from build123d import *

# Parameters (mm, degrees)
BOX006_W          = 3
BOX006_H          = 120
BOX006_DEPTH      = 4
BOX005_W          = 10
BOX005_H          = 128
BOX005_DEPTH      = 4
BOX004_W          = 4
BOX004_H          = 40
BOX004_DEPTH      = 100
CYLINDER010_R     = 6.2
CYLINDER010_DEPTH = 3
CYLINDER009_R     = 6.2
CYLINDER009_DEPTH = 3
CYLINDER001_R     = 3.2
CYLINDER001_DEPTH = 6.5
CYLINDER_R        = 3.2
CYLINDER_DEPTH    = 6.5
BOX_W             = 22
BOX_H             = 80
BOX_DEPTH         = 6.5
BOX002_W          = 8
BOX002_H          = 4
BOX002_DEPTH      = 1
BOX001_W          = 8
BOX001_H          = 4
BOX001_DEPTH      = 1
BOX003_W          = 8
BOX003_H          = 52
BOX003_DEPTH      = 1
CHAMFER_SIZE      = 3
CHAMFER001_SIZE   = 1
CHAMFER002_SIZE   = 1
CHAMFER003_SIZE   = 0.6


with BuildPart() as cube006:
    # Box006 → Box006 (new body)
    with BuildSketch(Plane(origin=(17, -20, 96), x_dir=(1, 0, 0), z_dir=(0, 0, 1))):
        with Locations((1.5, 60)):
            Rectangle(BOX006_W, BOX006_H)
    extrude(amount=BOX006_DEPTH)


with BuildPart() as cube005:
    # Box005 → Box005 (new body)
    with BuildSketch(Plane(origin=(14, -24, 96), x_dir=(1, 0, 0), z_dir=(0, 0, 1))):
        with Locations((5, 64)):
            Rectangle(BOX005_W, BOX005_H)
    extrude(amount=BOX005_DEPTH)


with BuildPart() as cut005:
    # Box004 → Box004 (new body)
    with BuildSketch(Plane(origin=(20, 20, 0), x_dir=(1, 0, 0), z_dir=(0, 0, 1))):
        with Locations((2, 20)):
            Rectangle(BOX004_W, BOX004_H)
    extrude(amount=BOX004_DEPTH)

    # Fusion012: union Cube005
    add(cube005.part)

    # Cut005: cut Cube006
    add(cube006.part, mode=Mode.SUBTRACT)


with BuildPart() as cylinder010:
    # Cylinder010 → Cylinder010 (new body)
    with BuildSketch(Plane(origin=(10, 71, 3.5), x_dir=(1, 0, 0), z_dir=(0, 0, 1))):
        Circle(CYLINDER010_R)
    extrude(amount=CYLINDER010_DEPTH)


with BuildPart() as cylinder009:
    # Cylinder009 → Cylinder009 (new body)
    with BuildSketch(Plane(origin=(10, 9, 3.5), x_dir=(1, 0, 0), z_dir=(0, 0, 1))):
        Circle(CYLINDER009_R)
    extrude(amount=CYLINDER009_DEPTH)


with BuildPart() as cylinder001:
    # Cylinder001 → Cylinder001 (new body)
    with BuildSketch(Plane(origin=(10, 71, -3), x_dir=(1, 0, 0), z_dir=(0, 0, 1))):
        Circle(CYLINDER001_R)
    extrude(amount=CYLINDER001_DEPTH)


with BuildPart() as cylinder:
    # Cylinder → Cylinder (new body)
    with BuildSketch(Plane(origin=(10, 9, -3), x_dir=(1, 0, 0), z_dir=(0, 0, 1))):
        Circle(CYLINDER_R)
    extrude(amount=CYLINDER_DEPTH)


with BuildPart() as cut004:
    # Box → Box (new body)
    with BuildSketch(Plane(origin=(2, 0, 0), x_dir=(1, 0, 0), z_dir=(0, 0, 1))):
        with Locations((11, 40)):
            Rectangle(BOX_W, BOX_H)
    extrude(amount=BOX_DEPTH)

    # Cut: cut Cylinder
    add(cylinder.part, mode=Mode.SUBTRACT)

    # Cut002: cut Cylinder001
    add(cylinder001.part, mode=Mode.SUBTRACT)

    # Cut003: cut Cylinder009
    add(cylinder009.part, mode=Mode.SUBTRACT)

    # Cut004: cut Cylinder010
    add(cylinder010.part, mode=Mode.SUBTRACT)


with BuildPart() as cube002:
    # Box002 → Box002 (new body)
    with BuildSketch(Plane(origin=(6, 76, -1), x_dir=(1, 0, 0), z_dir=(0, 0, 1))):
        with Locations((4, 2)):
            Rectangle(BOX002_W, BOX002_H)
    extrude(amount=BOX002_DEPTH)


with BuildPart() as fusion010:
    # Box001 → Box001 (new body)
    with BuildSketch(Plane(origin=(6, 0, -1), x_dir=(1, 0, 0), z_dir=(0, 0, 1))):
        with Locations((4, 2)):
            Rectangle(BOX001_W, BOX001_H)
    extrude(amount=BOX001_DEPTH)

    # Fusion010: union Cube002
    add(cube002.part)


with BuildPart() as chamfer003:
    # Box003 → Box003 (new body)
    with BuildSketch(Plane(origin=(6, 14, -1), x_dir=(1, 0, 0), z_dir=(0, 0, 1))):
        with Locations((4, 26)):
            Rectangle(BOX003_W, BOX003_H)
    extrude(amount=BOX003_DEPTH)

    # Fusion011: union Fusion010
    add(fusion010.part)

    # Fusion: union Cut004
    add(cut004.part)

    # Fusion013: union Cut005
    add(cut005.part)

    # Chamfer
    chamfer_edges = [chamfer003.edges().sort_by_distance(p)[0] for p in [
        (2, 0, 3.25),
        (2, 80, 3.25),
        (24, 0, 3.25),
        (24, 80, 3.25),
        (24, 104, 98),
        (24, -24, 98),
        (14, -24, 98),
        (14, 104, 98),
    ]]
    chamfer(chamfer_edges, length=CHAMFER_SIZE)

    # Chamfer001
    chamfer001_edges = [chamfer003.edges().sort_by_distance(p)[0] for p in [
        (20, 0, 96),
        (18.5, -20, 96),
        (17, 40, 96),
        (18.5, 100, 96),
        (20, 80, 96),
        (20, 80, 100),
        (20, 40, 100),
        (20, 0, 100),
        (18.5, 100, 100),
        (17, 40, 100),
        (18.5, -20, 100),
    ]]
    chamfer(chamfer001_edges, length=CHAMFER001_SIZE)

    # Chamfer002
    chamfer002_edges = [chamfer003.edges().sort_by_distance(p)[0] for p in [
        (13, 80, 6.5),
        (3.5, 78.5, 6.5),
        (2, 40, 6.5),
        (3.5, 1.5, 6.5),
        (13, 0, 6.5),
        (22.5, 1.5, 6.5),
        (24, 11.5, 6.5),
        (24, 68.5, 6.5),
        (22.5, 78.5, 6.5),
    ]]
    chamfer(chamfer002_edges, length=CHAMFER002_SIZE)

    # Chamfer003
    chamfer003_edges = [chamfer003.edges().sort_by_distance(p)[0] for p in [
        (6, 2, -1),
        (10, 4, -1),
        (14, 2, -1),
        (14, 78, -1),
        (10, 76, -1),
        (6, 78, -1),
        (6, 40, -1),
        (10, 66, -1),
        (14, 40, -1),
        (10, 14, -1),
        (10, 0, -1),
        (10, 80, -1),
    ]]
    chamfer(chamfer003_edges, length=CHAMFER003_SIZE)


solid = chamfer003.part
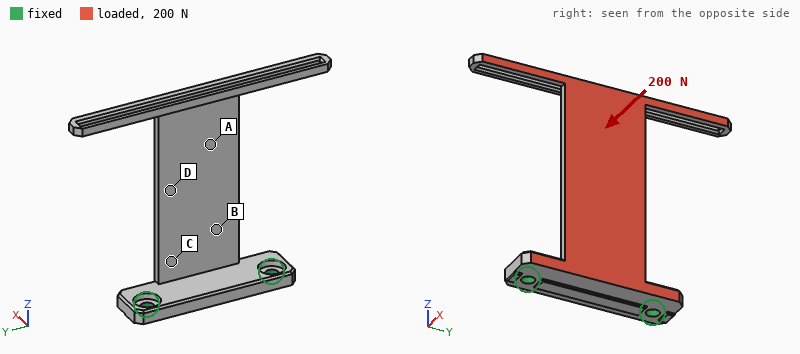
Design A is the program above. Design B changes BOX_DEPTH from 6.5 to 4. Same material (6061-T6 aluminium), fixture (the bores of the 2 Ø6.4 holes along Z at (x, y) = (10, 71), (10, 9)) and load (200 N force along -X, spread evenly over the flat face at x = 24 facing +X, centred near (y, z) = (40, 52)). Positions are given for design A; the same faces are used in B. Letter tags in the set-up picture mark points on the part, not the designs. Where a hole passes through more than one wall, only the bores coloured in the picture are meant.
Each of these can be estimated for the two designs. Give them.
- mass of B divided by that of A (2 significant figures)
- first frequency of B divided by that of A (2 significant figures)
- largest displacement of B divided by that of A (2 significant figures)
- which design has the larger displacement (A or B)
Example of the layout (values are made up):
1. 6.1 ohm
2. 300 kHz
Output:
1. 0.88
2. 0.87
3. 1.4
4. B
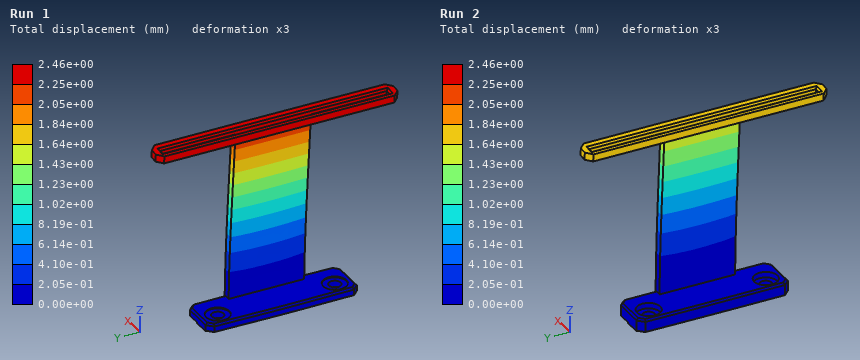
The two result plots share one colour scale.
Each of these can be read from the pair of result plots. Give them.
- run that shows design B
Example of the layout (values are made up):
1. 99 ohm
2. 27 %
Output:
1. Run 1
